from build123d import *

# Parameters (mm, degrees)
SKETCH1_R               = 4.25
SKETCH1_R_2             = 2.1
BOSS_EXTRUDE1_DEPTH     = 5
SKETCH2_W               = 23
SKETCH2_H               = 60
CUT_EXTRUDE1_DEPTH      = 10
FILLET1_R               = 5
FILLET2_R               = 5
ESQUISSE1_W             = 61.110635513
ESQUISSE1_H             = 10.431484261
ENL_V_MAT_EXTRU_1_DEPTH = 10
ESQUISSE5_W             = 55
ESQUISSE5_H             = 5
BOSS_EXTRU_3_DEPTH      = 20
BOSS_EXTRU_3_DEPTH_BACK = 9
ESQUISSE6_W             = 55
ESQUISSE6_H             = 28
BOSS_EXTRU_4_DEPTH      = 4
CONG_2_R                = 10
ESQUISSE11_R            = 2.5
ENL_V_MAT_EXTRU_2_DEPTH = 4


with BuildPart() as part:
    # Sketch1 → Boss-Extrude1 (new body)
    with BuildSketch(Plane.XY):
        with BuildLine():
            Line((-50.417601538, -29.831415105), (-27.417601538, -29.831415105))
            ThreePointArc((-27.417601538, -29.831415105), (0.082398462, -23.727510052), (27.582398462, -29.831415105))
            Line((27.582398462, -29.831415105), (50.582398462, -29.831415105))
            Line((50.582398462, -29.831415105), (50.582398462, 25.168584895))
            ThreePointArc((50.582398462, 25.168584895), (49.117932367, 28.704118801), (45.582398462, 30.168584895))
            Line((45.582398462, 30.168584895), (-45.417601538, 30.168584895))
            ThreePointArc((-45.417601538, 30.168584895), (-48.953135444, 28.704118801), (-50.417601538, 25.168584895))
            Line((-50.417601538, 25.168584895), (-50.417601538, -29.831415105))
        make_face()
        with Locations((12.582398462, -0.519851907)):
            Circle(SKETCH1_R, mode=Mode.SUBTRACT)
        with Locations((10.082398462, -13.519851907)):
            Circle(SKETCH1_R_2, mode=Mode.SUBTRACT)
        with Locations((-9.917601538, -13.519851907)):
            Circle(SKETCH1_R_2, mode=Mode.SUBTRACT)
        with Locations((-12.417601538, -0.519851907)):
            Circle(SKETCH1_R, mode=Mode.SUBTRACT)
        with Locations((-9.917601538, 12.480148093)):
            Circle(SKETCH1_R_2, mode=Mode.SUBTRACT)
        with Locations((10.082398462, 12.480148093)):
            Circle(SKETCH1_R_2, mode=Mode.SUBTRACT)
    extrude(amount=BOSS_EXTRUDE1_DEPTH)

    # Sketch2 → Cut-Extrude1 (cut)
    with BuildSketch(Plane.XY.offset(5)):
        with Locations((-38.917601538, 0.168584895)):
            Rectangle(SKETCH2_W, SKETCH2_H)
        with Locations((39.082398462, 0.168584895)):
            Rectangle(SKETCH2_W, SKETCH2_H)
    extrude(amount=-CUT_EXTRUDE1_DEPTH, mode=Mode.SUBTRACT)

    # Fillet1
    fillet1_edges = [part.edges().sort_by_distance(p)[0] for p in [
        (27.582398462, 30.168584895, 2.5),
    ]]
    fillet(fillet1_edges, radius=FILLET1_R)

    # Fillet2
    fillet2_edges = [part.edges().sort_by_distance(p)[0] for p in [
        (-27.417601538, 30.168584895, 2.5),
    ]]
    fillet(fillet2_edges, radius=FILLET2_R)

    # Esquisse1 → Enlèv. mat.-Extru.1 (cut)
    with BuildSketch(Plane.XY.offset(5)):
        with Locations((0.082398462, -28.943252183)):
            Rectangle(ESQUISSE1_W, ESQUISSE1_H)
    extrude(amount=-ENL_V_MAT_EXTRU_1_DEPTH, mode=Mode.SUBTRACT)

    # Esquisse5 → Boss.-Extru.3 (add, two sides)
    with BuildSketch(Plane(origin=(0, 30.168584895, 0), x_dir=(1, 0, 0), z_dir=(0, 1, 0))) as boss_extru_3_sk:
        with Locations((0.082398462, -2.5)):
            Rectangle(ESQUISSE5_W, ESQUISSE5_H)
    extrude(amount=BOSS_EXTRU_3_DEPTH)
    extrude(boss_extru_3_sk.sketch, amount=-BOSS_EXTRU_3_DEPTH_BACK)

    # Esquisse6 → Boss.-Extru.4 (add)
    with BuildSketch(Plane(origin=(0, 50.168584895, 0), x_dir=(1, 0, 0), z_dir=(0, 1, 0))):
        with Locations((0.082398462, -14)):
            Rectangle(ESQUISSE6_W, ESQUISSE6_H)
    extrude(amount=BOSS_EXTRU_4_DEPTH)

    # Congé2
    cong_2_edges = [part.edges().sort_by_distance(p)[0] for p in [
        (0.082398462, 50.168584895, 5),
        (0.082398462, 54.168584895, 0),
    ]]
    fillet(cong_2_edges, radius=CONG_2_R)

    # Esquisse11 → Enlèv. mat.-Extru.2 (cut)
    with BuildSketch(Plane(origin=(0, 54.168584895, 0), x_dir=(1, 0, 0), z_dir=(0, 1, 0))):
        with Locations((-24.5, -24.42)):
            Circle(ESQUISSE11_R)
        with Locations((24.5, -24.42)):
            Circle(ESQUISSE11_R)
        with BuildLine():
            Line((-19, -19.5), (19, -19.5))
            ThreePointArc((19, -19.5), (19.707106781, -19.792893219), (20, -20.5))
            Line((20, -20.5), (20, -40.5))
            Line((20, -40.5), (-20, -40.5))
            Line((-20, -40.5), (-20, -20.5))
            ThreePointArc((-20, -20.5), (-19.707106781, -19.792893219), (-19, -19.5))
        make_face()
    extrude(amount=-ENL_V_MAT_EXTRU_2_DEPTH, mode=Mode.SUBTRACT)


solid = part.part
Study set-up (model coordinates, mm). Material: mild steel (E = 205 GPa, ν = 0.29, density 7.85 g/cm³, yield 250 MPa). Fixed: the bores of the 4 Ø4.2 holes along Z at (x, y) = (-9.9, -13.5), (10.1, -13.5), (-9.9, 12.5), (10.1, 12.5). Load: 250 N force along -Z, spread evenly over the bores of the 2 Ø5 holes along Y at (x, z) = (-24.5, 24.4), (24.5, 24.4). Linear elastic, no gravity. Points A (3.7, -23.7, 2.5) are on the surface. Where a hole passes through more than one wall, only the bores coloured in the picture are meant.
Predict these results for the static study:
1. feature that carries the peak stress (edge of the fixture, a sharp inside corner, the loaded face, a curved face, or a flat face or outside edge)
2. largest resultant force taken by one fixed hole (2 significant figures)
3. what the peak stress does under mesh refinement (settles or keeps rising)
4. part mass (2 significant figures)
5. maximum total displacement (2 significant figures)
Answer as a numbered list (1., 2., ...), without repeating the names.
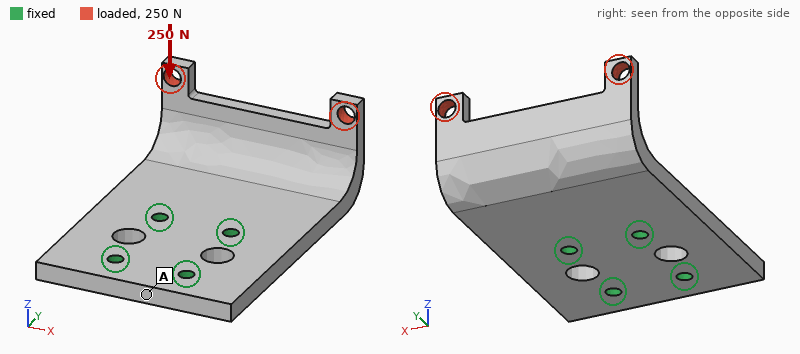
1. edge of the fixture
2. 190 N
3. keeps rising
4. 190 g
5. 66 µm
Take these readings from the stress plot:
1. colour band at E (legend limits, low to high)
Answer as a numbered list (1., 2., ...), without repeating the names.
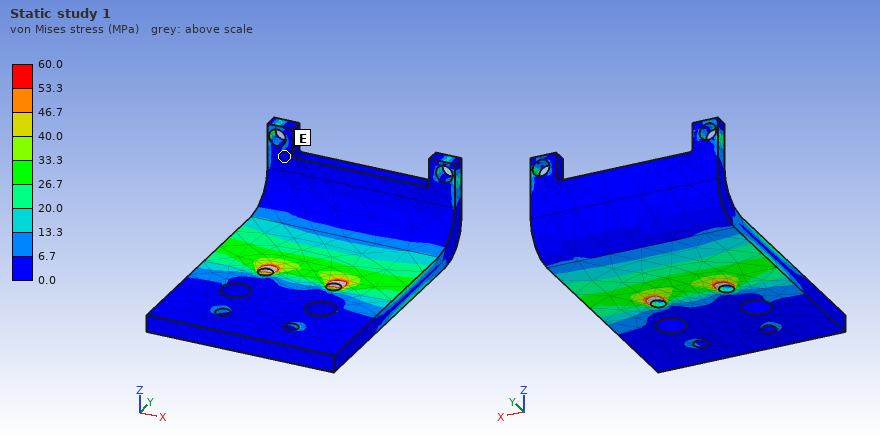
1. 0.0 to 6.7 MPa
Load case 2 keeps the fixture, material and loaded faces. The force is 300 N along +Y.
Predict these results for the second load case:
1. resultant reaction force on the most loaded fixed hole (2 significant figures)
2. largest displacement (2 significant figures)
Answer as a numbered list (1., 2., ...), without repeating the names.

1. 130 N
2. 88 µm
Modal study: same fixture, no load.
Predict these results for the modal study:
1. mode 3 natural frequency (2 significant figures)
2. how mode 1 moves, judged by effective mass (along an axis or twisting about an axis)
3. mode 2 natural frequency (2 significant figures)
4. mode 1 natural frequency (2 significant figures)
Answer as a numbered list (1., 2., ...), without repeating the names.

1. 7200 Hz
2. along Z
3. 2900 Hz
4. 1600 Hz
